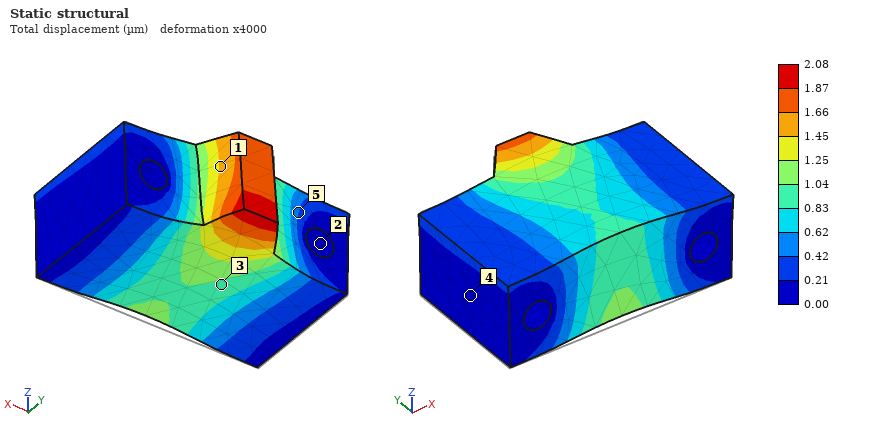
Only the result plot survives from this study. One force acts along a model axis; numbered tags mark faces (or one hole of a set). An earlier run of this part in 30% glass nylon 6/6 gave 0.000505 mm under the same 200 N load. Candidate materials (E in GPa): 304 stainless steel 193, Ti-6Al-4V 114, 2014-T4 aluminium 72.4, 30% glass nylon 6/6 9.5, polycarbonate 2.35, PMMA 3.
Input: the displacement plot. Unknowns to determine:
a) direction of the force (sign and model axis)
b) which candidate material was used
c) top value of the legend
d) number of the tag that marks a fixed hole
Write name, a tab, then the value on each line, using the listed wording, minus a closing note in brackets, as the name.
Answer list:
direction of the force	+Z
which candidate material was used	polycarbonate
top value of the legend	2.08 µm
number of the tag that marks a fixed hole	2
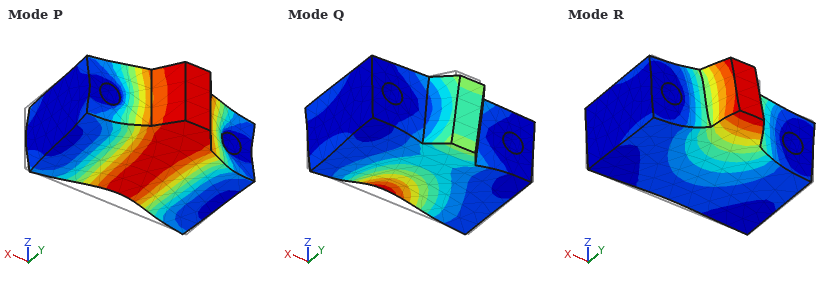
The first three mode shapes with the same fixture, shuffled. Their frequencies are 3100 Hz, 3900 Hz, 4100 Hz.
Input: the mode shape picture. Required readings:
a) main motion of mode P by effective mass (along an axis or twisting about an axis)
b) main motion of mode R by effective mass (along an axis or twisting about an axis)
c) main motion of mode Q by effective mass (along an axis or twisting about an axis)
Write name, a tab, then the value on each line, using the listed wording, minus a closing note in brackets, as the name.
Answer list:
main motion of mode P by effective mass	along Y
main motion of mode R by effective mass	along Z
main motion of mode Q by effective mass	along Z
